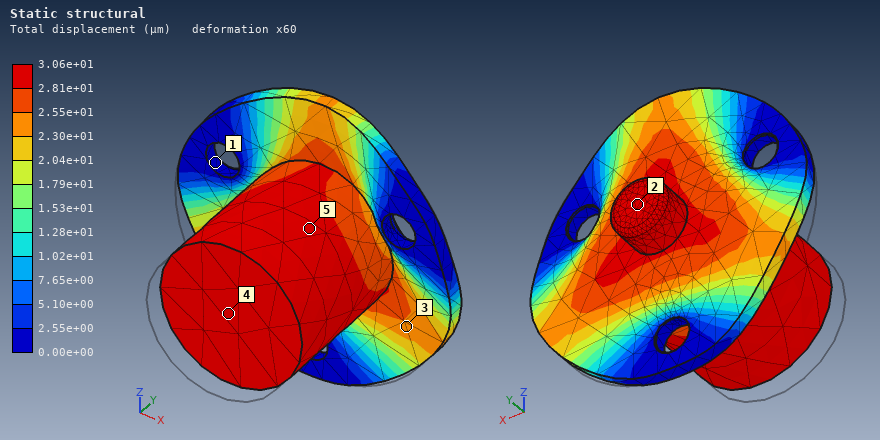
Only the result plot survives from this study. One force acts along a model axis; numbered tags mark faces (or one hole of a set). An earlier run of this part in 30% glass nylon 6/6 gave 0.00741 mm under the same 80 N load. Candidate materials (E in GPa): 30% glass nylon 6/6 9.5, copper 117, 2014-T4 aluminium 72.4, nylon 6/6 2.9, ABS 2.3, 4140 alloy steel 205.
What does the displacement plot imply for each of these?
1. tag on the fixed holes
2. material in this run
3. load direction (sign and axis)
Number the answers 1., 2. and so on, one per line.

1. 1
2. ABS
3. +Y
